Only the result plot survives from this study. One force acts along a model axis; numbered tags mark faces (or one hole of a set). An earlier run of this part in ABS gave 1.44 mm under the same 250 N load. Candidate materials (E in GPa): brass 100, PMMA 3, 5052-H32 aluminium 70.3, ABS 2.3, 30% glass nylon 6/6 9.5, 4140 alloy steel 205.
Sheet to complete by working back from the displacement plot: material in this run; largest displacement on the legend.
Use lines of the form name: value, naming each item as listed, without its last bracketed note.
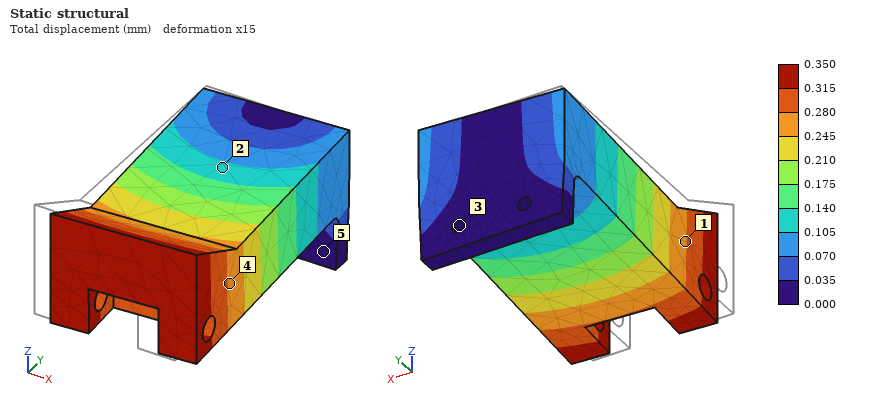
material in this run: 30% glass nylon 6/6
largest displacement on the legend: 0.350 mm
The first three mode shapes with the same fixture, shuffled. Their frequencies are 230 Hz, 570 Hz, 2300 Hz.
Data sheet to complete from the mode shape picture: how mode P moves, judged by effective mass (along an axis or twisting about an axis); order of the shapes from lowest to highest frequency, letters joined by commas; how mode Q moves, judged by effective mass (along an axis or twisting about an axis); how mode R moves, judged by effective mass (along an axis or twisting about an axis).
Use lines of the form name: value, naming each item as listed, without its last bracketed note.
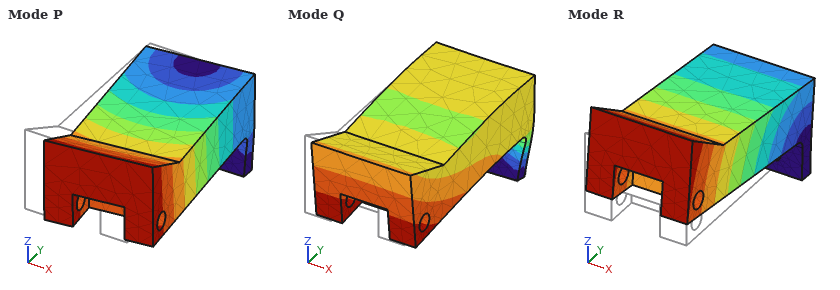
how mode P moves, judged by effective mass: along X
order of the shapes from lowest to highest frequency, letters joined by commas: R, P, Q
how mode Q moves, judged by effective mass: along Y
how mode R moves, judged by effective mass: along Z
